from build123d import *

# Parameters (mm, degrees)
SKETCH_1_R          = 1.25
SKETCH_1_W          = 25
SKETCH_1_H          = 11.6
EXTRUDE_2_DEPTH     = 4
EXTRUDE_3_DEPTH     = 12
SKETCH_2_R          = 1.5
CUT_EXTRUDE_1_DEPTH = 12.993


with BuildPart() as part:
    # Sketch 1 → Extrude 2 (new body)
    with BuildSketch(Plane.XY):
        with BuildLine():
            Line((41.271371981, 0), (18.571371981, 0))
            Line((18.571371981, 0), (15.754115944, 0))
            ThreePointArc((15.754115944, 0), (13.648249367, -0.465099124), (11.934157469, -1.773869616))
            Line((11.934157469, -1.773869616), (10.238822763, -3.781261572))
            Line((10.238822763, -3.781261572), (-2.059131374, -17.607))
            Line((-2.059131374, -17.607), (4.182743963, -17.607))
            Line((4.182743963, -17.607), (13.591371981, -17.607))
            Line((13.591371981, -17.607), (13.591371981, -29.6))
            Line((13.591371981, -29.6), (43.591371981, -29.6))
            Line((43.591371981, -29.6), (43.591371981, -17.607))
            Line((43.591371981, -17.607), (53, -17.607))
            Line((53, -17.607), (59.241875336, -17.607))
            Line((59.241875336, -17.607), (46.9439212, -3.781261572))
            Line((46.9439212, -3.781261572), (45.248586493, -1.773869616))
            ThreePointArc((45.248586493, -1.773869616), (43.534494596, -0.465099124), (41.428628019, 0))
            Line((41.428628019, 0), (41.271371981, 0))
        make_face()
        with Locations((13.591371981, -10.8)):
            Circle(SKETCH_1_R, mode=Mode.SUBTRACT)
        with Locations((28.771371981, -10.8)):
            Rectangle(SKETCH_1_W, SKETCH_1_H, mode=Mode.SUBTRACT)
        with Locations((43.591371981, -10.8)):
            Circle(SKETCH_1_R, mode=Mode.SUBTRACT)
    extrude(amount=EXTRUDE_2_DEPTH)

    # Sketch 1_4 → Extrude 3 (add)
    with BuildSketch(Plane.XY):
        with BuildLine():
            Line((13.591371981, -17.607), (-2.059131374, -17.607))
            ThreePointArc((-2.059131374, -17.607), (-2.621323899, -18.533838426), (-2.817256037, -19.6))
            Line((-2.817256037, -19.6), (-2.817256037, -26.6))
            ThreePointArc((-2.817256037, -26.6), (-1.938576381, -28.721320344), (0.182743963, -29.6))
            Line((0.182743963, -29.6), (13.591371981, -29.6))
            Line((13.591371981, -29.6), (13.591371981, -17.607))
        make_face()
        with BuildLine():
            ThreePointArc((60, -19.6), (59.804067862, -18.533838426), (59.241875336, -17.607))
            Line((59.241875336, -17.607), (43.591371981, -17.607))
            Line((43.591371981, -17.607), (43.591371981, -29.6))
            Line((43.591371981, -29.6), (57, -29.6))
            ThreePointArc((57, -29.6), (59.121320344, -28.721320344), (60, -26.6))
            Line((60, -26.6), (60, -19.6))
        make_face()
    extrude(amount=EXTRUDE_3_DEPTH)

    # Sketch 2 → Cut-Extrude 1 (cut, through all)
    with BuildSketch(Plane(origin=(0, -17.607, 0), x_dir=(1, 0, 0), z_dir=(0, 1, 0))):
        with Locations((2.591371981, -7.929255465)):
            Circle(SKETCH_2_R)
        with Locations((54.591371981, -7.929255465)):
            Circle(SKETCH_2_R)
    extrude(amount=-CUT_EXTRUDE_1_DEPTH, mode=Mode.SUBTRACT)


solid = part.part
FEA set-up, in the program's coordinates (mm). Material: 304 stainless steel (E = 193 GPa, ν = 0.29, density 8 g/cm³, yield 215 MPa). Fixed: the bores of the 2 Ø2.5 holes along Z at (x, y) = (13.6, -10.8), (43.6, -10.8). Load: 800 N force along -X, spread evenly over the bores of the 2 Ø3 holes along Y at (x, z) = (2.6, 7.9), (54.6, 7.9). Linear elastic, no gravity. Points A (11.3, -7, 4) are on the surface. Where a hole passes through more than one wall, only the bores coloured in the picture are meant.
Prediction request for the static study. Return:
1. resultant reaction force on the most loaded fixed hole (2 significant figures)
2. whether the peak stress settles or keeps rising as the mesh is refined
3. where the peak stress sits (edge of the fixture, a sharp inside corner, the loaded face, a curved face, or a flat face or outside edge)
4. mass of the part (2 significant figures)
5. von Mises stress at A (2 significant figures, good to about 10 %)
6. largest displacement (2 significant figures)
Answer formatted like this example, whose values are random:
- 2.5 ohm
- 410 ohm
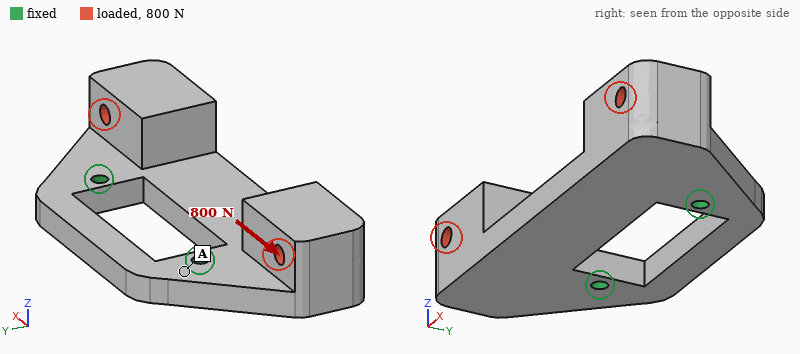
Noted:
- 480 N
- keeps rising
- edge of the fixture
- 64 g
- 14 MPa
- 20 µm
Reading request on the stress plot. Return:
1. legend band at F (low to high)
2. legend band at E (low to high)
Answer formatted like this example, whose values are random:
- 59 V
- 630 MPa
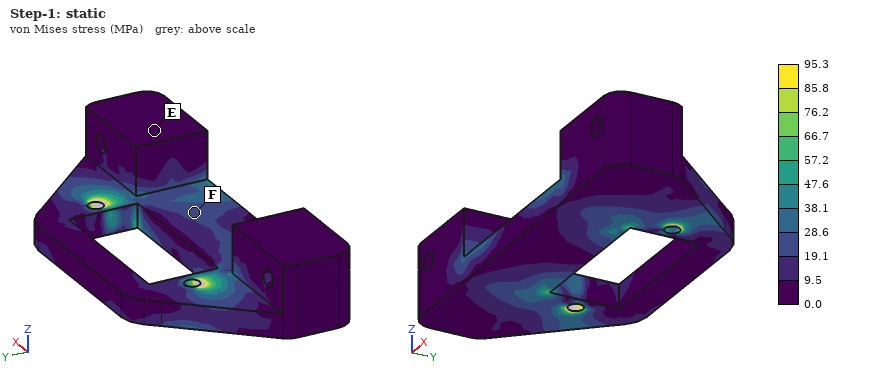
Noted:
- 19.1 to 28.6 MPa
- 0.0 to 9.5 MPa
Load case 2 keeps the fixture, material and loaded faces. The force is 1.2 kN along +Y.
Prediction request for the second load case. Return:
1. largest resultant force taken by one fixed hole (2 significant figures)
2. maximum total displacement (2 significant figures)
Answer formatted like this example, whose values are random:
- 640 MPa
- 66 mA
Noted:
- 660 N
- 49 µm
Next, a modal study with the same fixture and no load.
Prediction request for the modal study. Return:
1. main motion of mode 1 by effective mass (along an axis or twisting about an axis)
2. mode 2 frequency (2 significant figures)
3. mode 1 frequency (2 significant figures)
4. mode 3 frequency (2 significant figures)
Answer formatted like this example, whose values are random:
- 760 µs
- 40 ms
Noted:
- along Z
- 4000 Hz
- 3300 Hz
- 6200 Hz
